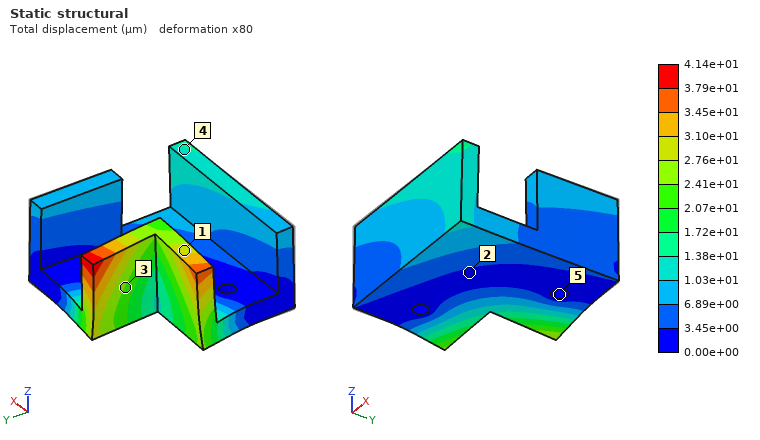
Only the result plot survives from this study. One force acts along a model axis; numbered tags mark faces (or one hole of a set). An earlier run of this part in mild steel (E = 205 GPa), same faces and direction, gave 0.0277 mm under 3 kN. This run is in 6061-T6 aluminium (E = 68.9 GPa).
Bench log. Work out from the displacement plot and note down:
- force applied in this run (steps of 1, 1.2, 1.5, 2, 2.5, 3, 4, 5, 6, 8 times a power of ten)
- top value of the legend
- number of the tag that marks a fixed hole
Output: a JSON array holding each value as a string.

["1.5 kN", "4.14e+01 µm", "5"]
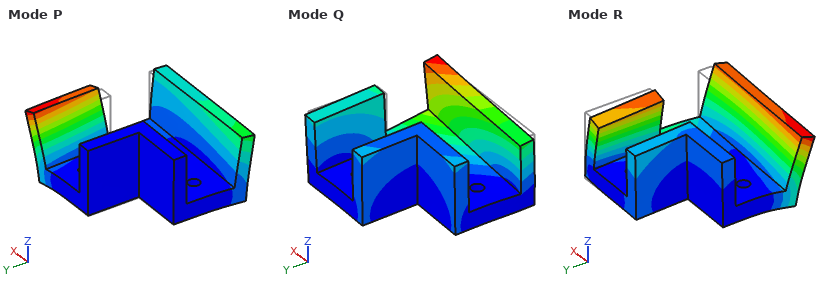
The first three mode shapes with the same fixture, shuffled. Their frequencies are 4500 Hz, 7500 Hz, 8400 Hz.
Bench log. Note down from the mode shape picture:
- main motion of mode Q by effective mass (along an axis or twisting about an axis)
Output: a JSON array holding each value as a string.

["along Z"]
